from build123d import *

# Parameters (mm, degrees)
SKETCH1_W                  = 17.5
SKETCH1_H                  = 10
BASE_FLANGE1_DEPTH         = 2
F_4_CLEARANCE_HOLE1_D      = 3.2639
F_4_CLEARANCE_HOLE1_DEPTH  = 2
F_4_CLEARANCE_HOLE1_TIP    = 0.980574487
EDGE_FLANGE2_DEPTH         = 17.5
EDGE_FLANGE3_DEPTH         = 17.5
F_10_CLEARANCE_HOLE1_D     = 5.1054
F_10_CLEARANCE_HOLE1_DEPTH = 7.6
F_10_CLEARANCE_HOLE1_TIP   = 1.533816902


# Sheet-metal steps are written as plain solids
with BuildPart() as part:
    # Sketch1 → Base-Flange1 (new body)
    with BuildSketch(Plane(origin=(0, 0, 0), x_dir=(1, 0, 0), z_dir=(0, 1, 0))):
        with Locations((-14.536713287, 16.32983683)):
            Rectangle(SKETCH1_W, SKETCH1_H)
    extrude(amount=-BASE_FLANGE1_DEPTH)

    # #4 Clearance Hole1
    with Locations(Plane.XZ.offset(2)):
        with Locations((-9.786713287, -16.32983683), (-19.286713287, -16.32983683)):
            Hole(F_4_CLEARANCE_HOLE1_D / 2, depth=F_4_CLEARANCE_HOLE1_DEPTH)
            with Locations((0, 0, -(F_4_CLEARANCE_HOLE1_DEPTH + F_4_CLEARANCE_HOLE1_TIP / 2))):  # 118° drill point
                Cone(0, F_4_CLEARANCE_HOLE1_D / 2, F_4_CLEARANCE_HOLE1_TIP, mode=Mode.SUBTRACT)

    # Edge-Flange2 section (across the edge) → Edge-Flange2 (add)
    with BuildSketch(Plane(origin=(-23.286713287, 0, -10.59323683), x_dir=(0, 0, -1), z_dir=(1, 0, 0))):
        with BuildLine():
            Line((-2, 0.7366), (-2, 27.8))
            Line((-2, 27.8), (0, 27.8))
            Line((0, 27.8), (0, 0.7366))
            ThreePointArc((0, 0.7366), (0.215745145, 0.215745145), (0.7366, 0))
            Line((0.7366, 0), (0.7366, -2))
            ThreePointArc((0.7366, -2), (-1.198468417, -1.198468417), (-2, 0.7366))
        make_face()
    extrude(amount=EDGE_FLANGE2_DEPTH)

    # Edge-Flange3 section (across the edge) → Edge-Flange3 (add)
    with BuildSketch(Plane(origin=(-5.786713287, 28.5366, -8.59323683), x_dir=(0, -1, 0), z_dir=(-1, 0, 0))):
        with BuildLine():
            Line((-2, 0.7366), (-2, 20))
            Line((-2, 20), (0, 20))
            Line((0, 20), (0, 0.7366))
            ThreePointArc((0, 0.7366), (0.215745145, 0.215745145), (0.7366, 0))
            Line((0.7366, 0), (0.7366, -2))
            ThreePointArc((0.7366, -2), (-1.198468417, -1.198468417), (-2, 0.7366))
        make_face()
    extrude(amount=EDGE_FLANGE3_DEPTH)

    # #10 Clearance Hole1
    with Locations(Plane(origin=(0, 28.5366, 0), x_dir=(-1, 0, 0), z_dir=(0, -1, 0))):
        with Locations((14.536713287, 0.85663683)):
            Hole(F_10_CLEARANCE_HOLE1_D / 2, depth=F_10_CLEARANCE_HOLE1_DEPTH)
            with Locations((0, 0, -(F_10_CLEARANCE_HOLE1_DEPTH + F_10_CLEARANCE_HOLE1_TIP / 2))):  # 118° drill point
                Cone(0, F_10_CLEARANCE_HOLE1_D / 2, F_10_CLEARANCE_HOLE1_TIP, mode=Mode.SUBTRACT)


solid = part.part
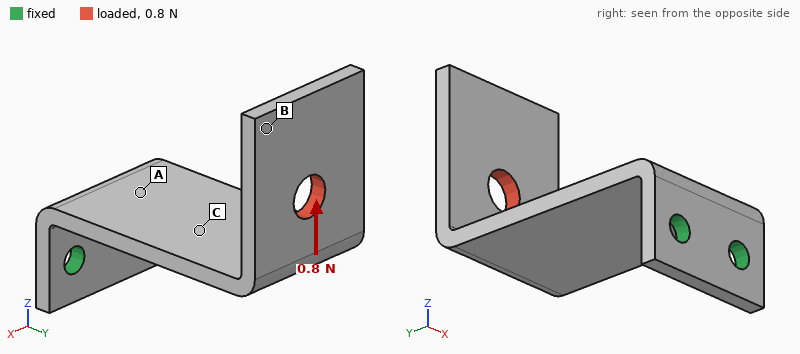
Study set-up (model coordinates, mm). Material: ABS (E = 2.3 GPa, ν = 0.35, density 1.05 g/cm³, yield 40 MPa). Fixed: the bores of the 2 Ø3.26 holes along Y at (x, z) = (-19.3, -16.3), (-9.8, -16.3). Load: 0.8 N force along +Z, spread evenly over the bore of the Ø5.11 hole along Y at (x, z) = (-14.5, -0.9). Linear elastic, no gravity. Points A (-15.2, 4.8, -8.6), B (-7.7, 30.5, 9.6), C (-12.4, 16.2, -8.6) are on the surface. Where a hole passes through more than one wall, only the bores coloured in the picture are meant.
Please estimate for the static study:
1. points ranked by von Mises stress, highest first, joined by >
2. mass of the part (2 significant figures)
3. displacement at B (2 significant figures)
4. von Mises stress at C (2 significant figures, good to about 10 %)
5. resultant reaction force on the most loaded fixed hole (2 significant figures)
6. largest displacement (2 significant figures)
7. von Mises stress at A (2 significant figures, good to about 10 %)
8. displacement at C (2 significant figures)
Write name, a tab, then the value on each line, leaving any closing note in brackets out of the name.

points ranked by von Mises stress, highest first, joined by >	A > C > B
mass of the part	2.2 g
displacement at B	0.54 mm
von Mises stress at C	0.87 MPa
resultant reaction force on the most loaded fixed hole	0.61 N
largest displacement	0.57 mm
von Mises stress at A	1.5 MPa
displacement at C	0.18 mm
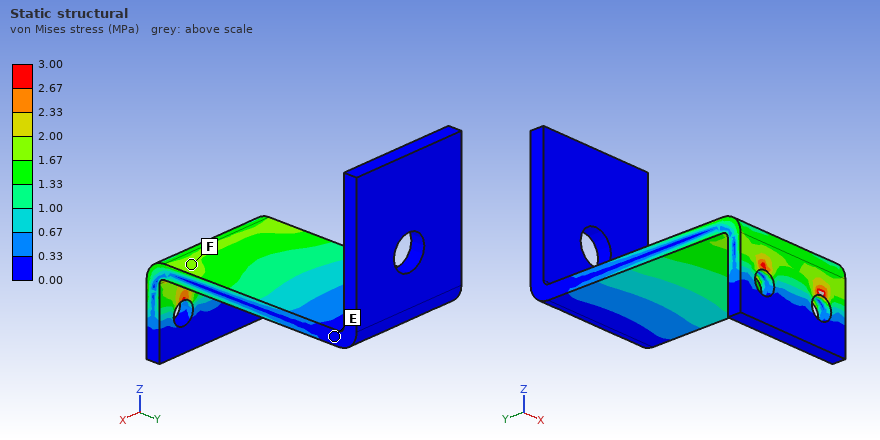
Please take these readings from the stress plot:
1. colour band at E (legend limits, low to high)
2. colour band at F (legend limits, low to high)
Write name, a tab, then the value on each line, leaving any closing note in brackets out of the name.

colour band at E	0.00 to 0.33 MPa
colour band at F	1.67 to 2.00 MPa
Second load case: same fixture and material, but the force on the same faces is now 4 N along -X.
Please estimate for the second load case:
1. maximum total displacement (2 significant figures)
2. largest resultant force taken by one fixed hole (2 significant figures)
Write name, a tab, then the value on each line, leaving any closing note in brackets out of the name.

maximum total displacement	0.59 mm
largest resultant force taken by one fixed hole	12 N
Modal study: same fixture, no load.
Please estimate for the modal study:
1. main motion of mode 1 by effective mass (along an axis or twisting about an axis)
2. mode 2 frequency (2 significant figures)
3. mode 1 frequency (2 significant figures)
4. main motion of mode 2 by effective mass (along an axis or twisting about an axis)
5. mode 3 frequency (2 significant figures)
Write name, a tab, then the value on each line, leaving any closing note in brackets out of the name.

main motion of mode 1 by effective mass	along Z
mode 2 frequency	500 Hz
mode 1 frequency	200 Hz
main motion of mode 2 by effective mass	along X
mode 3 frequency	740 Hz
